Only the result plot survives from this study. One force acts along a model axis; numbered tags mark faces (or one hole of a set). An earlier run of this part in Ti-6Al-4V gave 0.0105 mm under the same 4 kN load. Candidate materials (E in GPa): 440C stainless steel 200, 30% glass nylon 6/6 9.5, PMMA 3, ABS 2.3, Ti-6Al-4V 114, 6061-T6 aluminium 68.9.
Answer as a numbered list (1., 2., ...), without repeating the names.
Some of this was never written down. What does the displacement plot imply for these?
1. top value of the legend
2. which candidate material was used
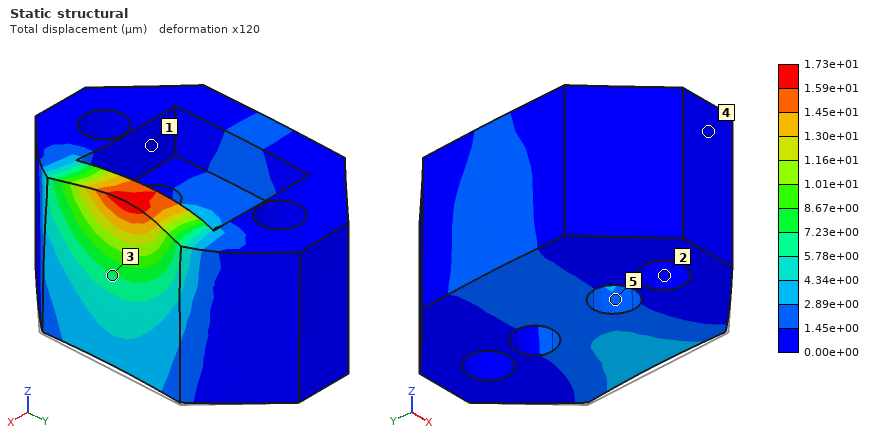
1. 1.73e+01 µm
2. 6061-T6 aluminium
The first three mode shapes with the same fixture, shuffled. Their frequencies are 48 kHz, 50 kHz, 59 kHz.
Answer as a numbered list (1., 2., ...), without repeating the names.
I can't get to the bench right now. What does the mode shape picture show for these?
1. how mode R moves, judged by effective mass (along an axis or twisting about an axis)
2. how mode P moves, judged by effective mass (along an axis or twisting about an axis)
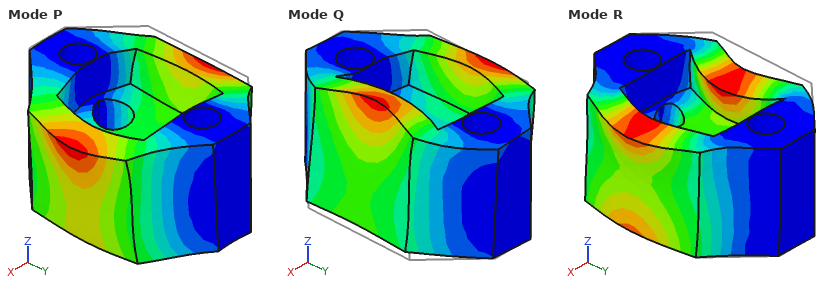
1. along X
2. along Z
